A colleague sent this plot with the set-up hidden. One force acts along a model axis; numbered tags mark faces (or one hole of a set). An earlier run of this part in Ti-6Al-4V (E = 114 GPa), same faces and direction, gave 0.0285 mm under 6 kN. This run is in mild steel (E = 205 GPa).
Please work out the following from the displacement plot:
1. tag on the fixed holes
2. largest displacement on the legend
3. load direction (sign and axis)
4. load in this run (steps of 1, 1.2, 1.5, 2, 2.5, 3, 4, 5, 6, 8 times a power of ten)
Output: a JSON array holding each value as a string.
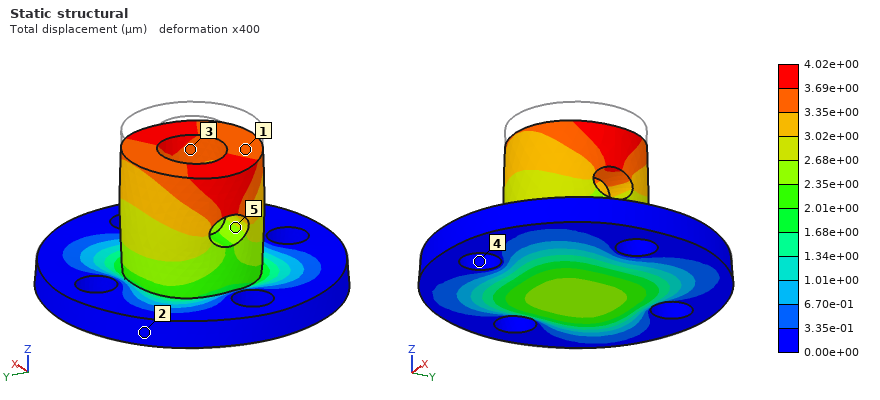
["4", "4.02e+00 µm", "-Z", "1.5 kN"]
